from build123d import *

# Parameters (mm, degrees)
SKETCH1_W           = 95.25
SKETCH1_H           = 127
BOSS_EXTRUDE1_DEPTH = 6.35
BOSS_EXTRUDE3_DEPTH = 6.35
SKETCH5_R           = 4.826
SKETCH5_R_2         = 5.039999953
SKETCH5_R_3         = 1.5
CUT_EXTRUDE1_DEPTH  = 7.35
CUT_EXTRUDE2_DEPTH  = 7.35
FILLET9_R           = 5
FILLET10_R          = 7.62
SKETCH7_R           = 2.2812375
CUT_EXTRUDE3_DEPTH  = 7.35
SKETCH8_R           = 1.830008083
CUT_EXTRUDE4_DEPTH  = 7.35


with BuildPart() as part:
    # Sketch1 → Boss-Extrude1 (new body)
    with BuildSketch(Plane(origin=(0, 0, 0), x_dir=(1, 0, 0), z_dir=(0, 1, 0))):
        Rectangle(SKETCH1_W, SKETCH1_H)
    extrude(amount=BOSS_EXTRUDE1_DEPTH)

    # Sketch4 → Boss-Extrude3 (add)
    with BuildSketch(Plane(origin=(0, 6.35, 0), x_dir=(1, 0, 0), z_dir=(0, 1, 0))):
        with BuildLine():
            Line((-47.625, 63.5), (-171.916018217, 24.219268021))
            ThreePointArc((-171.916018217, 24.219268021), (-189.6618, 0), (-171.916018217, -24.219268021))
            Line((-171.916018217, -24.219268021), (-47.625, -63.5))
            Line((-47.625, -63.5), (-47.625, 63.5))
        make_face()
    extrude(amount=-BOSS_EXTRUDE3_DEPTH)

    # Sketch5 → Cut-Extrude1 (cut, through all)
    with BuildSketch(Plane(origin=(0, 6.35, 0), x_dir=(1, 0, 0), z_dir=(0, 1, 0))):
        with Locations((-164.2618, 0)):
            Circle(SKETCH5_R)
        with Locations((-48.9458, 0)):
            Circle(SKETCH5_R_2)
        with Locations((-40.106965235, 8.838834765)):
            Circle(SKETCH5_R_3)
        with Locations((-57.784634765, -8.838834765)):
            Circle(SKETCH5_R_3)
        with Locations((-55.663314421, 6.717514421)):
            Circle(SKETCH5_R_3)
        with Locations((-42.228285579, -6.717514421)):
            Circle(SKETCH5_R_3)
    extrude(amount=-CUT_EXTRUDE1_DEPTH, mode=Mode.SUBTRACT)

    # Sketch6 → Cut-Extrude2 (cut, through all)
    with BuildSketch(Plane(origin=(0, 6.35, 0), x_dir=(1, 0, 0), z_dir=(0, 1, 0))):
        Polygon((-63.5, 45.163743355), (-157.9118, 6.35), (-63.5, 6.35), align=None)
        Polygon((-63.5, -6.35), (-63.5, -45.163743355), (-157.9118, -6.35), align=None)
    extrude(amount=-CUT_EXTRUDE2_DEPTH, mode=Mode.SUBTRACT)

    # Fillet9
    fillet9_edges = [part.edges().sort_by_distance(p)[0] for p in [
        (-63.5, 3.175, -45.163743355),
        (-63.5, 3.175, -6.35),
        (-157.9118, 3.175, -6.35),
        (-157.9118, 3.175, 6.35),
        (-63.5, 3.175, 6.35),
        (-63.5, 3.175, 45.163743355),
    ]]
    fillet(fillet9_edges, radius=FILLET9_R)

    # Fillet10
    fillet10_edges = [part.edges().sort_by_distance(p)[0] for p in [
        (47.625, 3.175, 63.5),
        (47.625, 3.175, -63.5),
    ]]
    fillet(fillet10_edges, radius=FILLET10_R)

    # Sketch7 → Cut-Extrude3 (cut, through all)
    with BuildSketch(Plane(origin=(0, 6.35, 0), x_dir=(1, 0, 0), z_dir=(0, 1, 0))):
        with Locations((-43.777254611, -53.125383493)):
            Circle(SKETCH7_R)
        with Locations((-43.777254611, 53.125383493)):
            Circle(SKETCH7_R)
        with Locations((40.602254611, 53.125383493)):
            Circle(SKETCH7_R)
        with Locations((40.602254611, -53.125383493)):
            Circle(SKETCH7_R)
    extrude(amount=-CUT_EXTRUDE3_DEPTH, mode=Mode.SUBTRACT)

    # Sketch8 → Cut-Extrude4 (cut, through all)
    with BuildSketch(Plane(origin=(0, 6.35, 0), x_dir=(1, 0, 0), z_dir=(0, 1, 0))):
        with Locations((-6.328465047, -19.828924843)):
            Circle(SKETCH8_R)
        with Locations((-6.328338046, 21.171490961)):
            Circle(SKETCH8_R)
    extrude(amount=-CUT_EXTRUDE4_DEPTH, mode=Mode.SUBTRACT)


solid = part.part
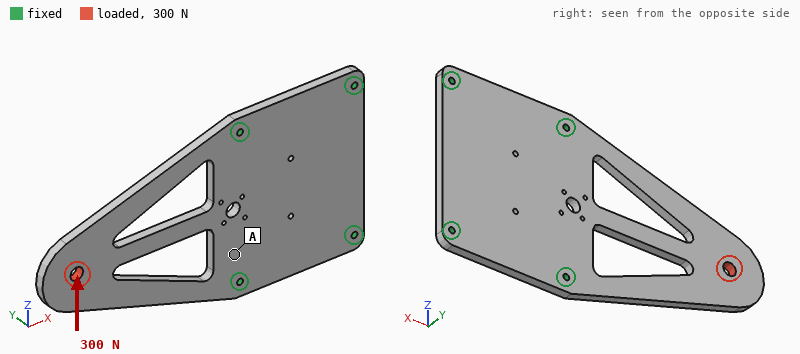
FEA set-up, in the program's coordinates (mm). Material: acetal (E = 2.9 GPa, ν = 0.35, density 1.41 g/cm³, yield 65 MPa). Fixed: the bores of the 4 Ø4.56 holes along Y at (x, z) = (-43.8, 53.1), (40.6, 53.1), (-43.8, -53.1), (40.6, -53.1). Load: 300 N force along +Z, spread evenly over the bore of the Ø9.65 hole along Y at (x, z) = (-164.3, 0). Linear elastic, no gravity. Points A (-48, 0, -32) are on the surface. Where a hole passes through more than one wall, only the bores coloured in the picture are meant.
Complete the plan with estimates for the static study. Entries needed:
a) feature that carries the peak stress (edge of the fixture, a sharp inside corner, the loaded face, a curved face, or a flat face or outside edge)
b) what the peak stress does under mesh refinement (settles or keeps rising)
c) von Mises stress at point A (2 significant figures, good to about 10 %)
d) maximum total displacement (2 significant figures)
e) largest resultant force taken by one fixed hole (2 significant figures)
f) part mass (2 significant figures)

a sharp inside corner
keeps rising
1.0 MPa
0.43 mm
350 N
180 g
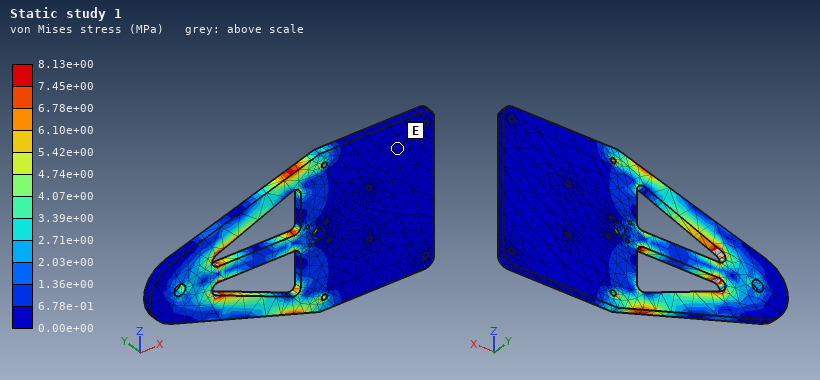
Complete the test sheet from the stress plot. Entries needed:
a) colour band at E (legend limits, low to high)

0.00e+00 to 6.78e-01 MPa
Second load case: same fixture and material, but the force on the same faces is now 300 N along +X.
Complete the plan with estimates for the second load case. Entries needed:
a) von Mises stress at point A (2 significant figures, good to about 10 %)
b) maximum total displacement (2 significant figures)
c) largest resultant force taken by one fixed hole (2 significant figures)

0.22 MPa
57 µm
130 N
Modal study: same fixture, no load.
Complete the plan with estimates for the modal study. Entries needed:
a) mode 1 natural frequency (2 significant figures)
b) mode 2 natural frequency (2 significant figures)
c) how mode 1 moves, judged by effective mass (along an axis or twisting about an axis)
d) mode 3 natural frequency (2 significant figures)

71 Hz
330 Hz
along Y
430 Hz
